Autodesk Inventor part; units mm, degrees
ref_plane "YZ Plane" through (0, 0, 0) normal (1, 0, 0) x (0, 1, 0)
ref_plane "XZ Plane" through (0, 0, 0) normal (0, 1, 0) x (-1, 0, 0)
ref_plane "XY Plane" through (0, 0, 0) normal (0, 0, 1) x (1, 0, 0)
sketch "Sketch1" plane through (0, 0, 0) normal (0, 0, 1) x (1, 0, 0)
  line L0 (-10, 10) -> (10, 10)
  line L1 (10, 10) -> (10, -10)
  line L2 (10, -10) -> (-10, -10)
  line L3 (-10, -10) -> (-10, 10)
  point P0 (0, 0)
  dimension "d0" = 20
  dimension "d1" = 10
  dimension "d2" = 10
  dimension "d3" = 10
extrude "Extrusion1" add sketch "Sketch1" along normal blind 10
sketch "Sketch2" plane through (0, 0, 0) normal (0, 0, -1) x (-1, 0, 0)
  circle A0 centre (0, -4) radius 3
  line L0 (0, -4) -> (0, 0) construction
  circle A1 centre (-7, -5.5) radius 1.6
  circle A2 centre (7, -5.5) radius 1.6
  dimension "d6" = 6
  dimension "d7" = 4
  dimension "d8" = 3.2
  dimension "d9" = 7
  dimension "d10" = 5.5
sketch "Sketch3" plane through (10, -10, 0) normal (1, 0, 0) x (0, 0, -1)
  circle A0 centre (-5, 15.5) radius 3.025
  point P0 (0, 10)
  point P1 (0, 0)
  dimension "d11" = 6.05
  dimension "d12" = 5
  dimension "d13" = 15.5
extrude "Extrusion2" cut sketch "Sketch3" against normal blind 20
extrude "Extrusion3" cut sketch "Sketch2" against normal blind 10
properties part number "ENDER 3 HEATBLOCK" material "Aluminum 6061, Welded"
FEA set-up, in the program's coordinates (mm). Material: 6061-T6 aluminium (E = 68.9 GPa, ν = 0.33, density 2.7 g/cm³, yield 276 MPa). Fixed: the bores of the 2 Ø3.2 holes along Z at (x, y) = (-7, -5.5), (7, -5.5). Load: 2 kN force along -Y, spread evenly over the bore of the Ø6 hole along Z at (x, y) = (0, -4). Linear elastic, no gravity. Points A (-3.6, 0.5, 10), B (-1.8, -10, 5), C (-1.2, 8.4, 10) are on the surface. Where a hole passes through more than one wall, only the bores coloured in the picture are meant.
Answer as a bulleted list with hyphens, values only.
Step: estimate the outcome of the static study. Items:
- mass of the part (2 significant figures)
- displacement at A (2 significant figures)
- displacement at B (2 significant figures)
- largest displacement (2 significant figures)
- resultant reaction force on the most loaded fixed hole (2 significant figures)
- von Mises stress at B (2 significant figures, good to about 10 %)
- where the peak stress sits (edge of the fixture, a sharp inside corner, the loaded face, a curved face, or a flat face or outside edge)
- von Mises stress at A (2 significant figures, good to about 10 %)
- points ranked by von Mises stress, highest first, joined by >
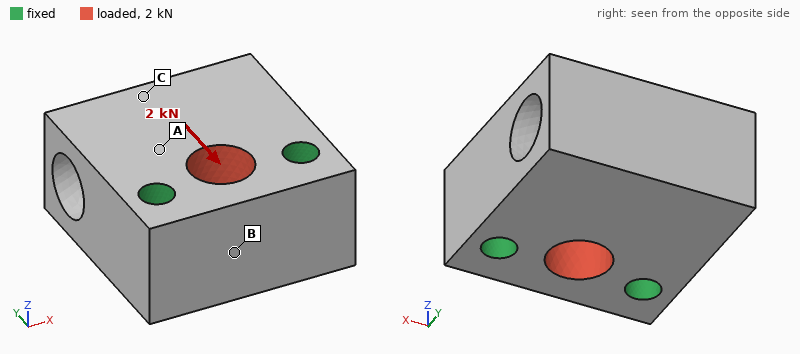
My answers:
- 8.0 g
- 1.1 µm
- 1.9 µm
- 2.7 µm
- 1.0 kN
- 16 MPa
- edge of the fixture
- 8.8 MPa
- B > A > C
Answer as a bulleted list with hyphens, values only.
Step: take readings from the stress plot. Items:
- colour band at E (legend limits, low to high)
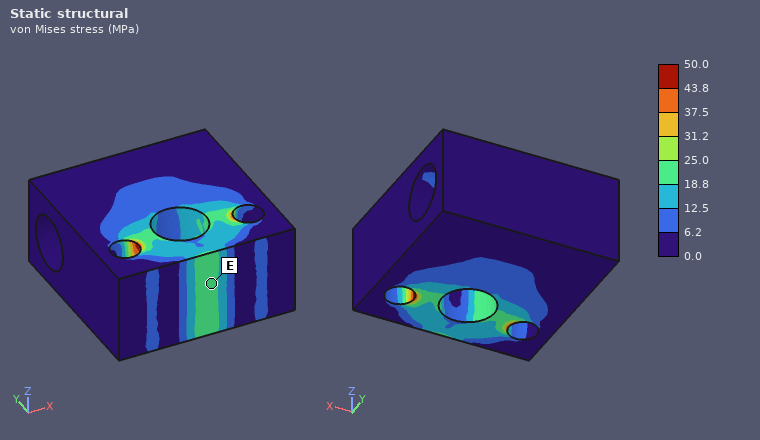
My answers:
- 18.8 to 25.0 MPa
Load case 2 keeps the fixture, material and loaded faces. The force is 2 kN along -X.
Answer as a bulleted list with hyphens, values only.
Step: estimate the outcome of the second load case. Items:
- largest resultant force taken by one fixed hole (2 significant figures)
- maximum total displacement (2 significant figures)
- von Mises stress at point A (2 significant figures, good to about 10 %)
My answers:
- 1.0 kN
- 1.9 µm
- 3.9 MPa
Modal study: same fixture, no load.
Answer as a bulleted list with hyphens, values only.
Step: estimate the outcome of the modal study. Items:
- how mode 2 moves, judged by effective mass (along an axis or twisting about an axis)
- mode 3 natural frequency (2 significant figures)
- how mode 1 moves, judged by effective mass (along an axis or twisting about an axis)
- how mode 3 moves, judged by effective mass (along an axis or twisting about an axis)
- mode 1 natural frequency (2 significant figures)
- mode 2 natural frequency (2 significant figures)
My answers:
- along X
- 41 kHz
- along Z
- twisting about Y
- 25 kHz
- 39 kHz
